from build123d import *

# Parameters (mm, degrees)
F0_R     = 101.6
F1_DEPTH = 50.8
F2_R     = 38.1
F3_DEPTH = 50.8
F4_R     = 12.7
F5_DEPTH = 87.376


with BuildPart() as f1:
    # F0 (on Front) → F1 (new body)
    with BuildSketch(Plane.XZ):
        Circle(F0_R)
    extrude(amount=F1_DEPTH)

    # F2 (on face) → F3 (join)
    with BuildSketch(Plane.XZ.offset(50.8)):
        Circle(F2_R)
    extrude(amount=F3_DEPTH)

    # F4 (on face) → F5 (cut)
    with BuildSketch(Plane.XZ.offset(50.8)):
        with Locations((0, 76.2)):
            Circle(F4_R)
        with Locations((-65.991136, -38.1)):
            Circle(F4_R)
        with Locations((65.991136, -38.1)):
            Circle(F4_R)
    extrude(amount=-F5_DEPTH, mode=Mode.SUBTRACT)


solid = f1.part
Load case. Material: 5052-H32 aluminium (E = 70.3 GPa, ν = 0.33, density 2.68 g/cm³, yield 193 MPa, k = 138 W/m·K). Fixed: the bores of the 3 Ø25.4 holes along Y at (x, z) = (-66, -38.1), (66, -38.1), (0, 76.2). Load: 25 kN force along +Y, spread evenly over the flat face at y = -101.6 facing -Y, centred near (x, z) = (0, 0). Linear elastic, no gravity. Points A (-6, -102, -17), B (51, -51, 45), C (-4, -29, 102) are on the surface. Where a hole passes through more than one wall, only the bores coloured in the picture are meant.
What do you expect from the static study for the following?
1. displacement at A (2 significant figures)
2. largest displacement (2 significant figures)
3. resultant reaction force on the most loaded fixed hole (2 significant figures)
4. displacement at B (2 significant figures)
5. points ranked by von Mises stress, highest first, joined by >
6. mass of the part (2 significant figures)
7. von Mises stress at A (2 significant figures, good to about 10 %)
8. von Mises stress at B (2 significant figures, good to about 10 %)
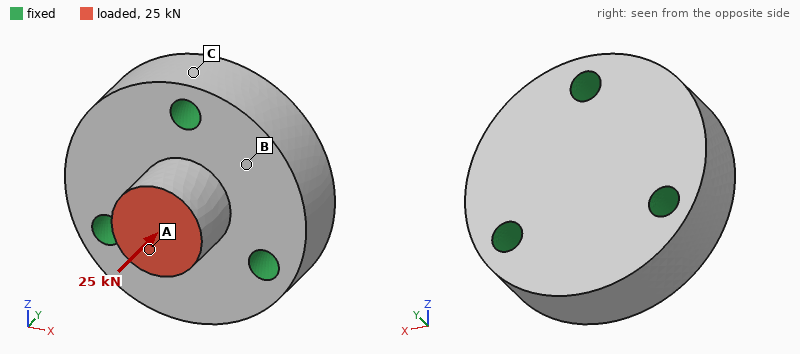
9.4 µm
9.5 µm
8.5 kN
2.5 µm
A > B > C
4.8 kg
5.6 MPa
1.7 MPa
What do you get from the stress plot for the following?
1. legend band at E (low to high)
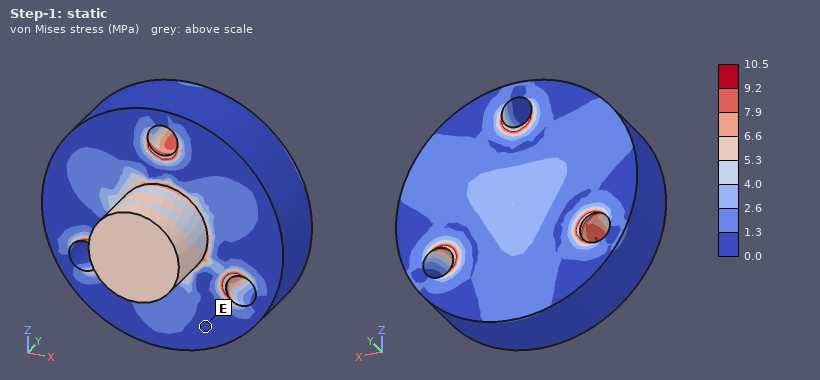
0.0 to 1.3 MPa
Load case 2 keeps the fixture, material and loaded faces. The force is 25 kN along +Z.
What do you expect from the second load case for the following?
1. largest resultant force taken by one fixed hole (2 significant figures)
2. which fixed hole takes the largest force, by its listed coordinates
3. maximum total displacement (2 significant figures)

18 kN
(0, 76.2)
47 µm
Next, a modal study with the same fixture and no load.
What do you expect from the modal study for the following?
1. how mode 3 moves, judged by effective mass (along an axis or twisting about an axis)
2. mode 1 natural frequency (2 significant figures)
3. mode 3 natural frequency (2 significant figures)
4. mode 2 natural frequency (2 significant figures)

along Y
6400 Hz
7100 Hz
6400 Hz
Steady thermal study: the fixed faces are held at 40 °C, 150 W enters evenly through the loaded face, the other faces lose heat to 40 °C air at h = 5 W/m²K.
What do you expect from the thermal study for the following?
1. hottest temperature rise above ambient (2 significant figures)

19 K
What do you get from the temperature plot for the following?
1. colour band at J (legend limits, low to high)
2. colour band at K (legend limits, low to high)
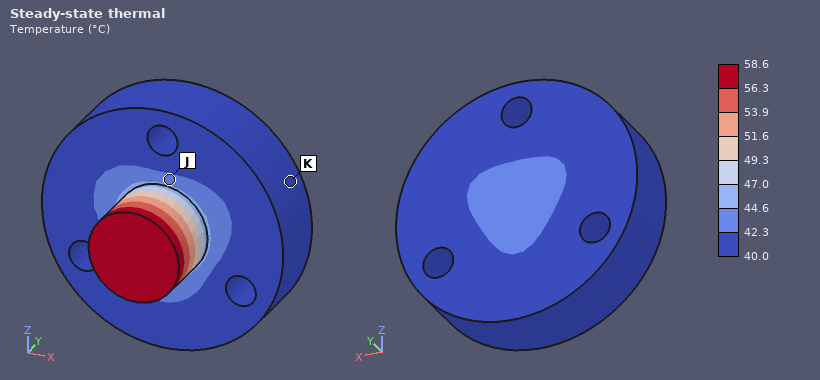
42.3 to 44.6 °C
40.0 to 42.3 °C
